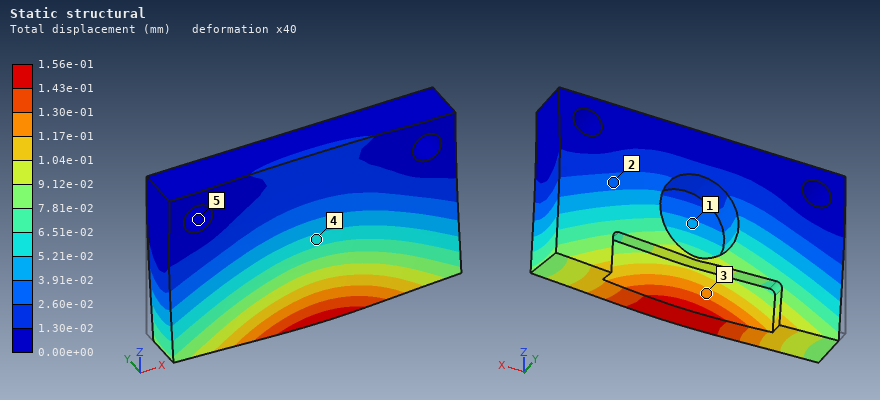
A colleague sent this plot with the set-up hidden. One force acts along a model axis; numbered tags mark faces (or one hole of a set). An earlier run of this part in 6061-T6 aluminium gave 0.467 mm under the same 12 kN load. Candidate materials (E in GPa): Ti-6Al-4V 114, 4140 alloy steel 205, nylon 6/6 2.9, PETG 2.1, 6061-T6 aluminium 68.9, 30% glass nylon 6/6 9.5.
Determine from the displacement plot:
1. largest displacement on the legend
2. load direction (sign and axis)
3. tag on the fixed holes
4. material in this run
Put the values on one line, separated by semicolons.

1.56e-01 mm; -Y; 5; 4140 alloy steel
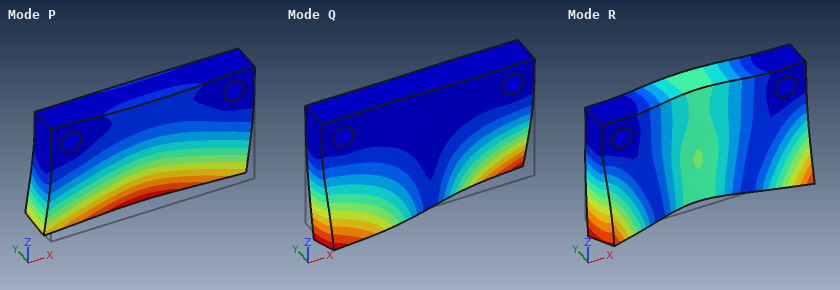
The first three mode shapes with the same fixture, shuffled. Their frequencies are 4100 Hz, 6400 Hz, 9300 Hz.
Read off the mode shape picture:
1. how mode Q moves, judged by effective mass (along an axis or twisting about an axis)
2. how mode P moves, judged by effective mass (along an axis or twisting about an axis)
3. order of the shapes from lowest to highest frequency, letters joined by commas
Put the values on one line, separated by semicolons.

twisting about Z; along Y; P, Q, R
